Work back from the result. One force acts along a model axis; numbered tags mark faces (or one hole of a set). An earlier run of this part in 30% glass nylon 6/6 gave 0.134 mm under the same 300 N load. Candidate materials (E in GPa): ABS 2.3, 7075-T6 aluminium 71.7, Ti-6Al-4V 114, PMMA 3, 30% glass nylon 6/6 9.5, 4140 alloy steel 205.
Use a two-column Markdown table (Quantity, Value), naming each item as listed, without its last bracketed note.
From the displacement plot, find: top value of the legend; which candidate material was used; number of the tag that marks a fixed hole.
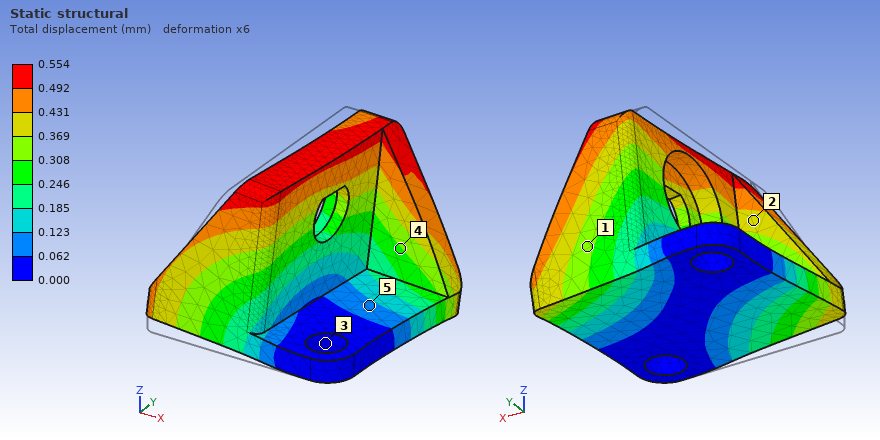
| Quantity | Value |
|---|---|
| top value of the legend | 0.554 mm |
| which candidate material was used | ABS |
| number of the tag that marks a fixed hole | 3 |
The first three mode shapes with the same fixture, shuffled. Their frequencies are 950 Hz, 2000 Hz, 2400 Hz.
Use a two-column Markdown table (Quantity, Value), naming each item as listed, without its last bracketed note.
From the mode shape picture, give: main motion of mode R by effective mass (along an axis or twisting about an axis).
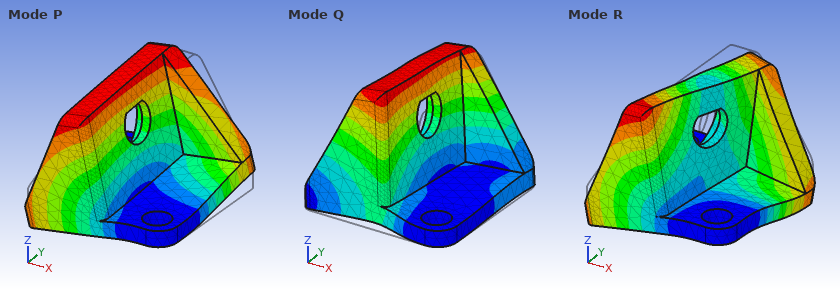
| Quantity | Value |
|---|---|
| main motion of mode R by effective mass | along Z |
